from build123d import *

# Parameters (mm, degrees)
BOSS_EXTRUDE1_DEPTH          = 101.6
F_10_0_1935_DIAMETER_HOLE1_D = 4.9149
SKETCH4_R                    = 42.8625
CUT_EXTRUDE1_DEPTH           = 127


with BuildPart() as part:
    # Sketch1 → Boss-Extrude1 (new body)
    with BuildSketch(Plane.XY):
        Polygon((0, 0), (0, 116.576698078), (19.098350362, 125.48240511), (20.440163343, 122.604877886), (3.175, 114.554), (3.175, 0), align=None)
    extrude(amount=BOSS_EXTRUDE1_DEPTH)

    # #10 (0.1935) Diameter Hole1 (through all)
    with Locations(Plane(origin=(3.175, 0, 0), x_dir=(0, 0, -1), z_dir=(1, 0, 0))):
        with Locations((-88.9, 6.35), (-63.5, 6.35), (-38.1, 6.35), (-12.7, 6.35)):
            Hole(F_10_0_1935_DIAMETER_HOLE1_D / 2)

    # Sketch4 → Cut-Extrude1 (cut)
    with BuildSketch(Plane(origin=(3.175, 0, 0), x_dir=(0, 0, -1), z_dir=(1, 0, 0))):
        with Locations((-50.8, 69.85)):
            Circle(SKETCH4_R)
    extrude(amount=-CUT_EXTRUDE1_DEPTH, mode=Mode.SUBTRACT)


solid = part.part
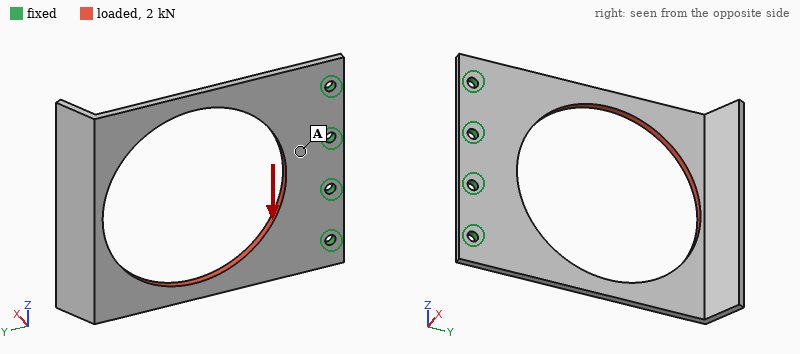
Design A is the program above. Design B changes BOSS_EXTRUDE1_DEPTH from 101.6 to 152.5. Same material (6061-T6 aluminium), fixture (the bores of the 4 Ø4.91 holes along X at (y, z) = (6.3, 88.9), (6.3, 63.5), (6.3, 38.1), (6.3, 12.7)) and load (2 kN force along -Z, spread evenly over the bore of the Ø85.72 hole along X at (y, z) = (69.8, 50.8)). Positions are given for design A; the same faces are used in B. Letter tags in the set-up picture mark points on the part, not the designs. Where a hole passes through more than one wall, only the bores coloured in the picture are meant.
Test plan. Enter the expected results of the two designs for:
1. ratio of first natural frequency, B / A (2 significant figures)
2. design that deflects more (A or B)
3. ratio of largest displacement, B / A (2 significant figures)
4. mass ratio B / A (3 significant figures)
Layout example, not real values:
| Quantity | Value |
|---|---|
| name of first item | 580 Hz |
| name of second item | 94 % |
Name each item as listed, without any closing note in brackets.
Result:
| Quantity | Value |
|---|---|
| ratio of first natural frequency, B / A | 1.0 |
| design that deflects more | A |
| ratio of largest displacement, B / A | 0.51 |
| mass ratio B / A | 1.87 |
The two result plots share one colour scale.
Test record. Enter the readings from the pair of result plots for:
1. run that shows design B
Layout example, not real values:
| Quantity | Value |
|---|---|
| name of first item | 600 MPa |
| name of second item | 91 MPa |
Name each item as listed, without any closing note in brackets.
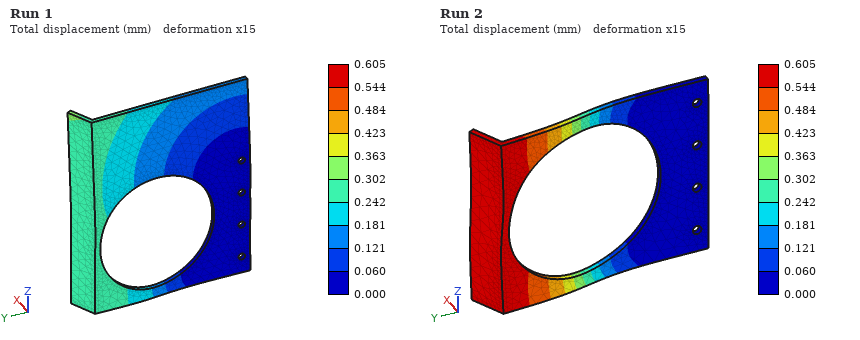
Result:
| Quantity | Value |
|---|---|
| run that shows design B | Run 1 |
